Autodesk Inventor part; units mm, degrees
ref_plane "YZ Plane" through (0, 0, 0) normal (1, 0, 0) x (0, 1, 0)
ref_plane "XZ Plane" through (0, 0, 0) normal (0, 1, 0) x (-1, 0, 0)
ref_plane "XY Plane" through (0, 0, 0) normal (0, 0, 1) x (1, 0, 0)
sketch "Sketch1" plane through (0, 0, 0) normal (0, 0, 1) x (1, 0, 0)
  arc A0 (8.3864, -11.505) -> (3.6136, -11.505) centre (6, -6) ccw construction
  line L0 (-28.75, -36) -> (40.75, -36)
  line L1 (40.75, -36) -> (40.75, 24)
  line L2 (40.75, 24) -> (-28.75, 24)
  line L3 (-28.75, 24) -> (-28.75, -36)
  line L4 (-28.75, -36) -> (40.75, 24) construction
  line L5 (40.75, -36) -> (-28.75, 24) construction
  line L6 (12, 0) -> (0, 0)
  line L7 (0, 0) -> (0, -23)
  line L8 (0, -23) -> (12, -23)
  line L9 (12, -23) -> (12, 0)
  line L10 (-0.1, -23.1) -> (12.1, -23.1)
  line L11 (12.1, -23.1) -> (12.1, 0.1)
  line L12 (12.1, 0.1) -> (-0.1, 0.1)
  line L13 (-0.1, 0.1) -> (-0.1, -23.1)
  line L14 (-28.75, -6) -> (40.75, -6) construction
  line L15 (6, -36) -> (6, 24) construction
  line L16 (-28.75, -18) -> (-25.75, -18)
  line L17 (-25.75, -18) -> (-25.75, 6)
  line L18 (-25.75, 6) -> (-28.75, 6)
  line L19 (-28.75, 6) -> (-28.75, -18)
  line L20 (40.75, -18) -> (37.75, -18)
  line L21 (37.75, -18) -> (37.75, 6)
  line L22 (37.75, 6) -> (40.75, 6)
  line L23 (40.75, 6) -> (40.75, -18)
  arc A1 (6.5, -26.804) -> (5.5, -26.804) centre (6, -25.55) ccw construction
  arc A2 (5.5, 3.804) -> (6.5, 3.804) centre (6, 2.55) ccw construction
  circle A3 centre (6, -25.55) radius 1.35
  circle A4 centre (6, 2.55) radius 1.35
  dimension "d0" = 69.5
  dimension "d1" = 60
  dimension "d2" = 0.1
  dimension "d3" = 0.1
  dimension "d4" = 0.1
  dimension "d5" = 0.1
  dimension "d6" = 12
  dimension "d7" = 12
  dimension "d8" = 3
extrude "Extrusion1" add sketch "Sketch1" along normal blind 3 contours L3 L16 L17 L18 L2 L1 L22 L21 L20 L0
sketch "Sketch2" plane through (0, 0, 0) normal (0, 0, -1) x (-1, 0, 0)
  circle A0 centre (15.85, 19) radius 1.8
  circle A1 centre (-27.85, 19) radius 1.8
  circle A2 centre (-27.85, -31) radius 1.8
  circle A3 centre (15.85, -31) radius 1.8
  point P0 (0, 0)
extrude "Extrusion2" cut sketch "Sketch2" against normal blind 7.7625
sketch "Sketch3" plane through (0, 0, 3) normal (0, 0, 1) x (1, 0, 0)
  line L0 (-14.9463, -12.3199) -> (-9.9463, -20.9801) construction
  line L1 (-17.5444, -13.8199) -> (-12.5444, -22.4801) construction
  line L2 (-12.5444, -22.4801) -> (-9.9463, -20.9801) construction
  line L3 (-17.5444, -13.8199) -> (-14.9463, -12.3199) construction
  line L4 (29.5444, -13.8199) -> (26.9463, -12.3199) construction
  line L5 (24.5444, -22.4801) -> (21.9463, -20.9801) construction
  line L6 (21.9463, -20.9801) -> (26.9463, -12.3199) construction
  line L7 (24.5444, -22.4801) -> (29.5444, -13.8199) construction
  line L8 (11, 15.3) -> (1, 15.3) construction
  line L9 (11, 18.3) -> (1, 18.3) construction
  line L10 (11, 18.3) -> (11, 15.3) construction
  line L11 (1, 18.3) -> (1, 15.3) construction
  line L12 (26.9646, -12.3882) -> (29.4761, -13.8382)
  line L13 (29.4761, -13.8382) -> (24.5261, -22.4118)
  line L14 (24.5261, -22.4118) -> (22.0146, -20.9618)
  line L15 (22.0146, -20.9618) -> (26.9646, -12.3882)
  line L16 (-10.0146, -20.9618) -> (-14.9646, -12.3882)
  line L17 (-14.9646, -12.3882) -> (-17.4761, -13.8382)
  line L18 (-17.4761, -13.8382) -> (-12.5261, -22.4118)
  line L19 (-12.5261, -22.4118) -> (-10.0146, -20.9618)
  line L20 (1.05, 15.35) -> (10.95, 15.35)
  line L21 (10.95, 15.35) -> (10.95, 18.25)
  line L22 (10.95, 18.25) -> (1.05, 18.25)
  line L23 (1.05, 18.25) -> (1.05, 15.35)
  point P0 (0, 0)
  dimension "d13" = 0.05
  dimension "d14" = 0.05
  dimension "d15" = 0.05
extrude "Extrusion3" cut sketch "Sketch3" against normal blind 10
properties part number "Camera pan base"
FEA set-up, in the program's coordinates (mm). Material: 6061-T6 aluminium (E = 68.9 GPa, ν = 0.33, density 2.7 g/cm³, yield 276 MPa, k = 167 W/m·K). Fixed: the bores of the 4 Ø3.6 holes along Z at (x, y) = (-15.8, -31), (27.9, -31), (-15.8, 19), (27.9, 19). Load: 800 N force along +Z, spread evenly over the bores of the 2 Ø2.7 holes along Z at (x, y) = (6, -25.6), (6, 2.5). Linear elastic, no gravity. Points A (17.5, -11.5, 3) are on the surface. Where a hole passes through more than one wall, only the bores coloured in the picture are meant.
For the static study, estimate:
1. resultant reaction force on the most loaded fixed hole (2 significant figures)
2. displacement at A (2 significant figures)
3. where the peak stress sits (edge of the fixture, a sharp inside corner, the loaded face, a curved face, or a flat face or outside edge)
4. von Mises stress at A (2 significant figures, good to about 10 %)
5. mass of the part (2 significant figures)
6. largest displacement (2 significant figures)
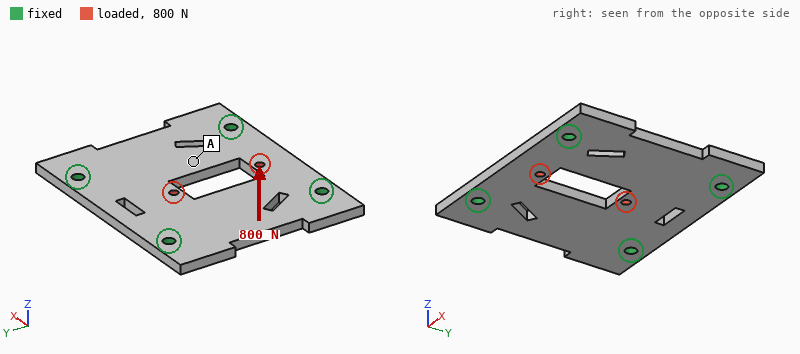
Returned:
240 N
0.089 mm
the loaded face
22 MPa
29 g
0.15 mm
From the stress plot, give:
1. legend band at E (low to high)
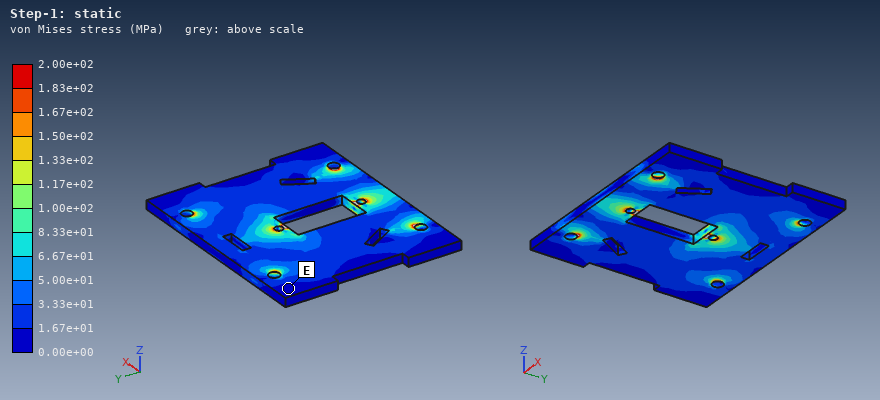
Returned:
0.00e+00 to 1.67e+01 MPa
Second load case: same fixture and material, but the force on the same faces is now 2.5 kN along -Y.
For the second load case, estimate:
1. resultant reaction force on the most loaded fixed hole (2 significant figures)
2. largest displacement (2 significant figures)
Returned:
770 N
22 µm
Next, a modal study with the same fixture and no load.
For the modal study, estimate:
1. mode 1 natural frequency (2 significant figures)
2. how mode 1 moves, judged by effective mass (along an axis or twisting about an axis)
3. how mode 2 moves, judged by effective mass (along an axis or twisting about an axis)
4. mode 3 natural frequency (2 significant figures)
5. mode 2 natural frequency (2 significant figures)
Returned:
5000 Hz
along Z
twisting about Y
6900 Hz
6400 Hz
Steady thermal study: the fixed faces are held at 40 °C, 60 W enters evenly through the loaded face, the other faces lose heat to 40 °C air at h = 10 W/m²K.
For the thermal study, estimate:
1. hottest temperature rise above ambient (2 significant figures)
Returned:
60 K
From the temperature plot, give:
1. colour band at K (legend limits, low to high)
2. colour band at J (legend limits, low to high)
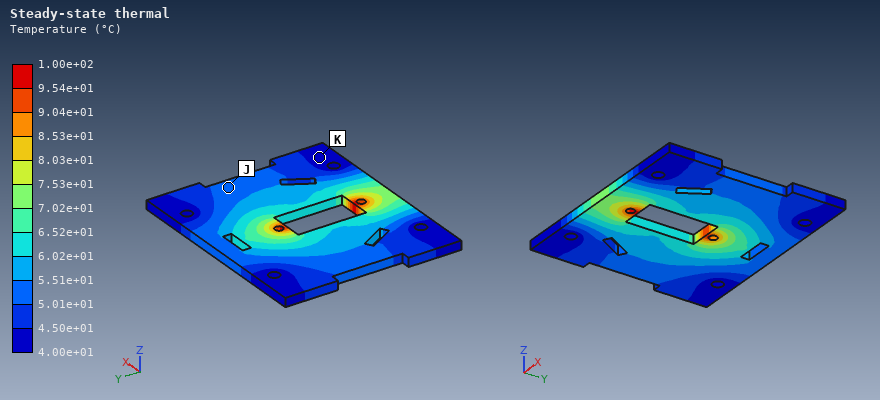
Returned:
4.00e+01 to 4.50e+01 °C
5.01e+01 to 5.51e+01 °C
